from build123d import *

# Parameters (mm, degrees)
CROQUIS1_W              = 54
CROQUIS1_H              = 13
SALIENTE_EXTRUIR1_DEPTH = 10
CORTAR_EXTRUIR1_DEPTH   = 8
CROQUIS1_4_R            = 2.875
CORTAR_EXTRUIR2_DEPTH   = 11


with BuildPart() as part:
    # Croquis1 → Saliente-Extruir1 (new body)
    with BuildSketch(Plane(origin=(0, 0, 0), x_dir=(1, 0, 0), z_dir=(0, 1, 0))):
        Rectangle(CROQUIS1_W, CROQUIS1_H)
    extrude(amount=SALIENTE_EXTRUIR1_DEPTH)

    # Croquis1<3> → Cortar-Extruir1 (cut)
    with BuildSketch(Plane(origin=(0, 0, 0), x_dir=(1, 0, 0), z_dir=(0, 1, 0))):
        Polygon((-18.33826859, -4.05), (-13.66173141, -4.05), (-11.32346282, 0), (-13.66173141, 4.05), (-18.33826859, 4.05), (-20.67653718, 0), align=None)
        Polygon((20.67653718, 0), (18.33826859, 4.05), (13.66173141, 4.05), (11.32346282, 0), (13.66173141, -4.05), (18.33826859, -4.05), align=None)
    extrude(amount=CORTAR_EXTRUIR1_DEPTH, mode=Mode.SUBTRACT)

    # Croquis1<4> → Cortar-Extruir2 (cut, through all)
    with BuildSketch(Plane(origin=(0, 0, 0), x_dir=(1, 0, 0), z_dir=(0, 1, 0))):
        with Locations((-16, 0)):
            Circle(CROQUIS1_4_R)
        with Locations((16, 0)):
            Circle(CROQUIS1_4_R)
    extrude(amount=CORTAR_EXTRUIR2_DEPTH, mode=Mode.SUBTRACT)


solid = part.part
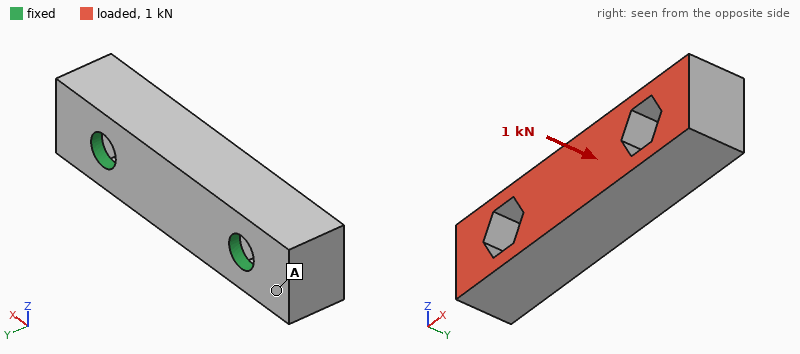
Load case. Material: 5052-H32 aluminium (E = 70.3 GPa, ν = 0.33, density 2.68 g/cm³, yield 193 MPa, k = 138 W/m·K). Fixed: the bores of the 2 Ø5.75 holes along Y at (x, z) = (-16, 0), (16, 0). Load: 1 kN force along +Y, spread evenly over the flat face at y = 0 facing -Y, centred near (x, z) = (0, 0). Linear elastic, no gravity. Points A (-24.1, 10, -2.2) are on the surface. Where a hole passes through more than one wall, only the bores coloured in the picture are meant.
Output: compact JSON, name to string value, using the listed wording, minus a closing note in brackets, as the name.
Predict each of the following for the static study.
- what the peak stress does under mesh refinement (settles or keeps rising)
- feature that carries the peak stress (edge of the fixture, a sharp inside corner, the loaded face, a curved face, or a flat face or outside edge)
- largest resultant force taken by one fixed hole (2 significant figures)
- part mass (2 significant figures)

{"what the peak stress does under mesh refinement": "keeps rising", "feature that carries the peak stress": "edge of the fixture", "largest resultant force taken by one fixed hole": "510 N", "part mass": "16 g"}
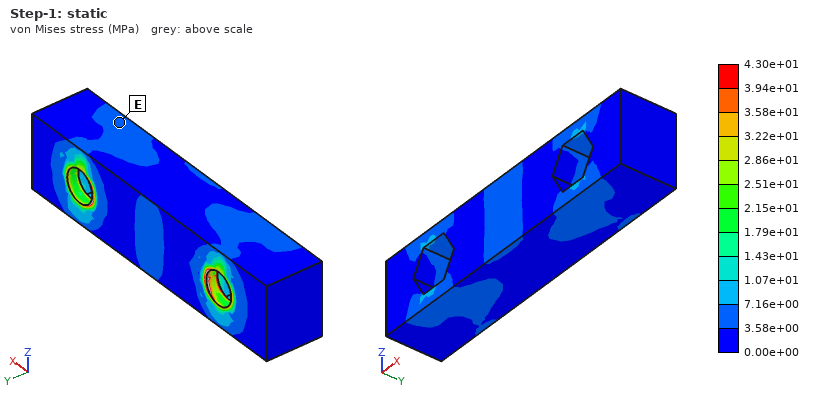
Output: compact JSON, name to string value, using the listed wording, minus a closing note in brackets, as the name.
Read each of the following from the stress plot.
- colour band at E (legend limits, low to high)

{"colour band at E": "3.58e+00 to 7.16e+00 MPa"}
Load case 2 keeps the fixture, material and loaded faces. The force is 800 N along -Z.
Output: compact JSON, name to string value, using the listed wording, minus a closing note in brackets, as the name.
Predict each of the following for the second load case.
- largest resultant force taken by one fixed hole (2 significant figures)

{"largest resultant force taken by one fixed hole": "400 N"}
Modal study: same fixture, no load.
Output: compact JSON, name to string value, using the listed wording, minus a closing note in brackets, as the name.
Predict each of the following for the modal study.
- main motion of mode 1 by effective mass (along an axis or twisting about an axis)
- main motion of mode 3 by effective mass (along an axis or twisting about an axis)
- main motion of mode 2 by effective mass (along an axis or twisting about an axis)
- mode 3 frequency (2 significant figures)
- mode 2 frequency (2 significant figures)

{"main motion of mode 1 by effective mass": "along Z", "main motion of mode 3 by effective mass": "along Y", "main motion of mode 2 by effective mass": "twisting about Y", "mode 3 frequency": "23 kHz", "mode 2 frequency": "21 kHz"}
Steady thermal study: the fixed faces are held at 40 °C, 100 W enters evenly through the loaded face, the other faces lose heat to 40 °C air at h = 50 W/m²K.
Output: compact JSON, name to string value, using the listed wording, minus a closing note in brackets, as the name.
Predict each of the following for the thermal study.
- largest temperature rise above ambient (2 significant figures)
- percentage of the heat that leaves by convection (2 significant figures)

{"largest temperature rise above ambient": "38 K", "percentage of the heat that leaves by convection": "3.0 %"}
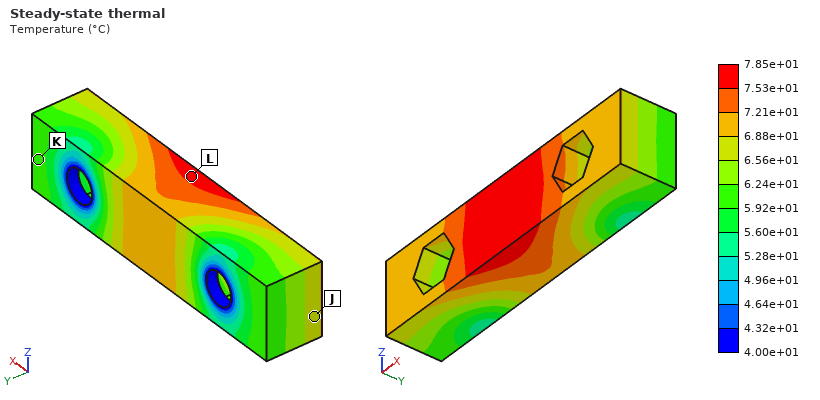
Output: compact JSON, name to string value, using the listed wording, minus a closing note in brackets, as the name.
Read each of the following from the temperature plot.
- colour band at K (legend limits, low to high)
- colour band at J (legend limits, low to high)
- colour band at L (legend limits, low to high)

{"colour band at K": "5.92e+01 to 6.24e+01 °C", "colour band at J": "6.56e+01 to 6.88e+01 °C", "colour band at L": "7.53e+01 to 7.85e+01 °C"}
